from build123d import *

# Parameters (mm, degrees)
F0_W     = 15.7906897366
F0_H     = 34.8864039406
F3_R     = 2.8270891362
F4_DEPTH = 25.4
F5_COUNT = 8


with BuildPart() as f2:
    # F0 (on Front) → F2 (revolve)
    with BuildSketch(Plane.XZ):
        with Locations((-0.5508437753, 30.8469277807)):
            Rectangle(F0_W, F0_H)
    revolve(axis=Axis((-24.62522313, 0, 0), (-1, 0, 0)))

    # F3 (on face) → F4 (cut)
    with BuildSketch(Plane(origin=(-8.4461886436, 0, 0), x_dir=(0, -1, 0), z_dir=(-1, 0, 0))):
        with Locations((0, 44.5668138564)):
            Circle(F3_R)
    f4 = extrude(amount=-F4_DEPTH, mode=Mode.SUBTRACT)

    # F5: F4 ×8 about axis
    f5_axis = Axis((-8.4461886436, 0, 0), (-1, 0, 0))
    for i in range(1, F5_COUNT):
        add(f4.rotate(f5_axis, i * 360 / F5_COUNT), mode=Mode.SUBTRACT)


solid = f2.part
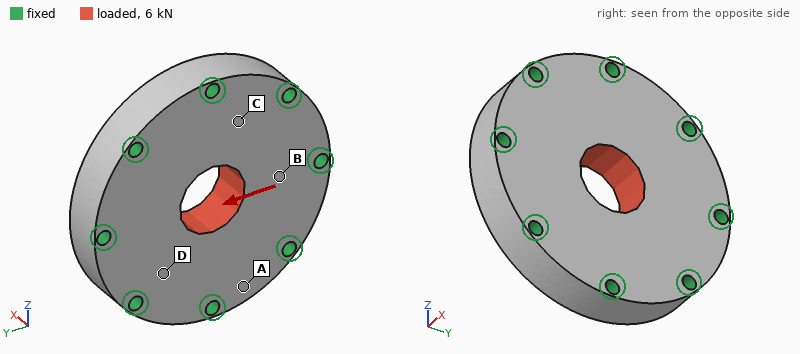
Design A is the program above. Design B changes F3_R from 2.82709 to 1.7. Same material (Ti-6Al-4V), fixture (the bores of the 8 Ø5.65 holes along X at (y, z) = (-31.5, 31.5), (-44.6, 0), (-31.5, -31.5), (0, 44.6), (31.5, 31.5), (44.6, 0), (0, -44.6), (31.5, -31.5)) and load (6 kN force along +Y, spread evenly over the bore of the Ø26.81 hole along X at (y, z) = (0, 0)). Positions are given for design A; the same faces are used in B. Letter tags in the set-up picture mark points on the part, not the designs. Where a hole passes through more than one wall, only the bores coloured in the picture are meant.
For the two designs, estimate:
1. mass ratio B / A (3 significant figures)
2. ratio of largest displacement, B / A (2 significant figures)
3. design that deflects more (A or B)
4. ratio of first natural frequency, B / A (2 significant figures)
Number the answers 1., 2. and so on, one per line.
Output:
1. 1.02
2. 1.1
3. B
4. 0.90
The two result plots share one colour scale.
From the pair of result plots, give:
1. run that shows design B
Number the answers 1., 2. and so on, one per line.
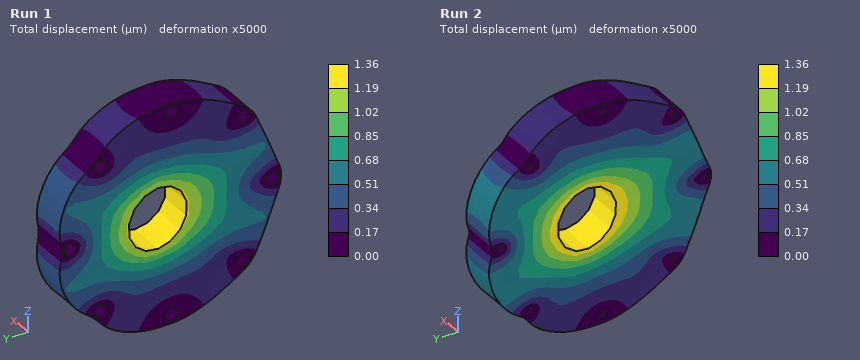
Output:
1. Run 2
